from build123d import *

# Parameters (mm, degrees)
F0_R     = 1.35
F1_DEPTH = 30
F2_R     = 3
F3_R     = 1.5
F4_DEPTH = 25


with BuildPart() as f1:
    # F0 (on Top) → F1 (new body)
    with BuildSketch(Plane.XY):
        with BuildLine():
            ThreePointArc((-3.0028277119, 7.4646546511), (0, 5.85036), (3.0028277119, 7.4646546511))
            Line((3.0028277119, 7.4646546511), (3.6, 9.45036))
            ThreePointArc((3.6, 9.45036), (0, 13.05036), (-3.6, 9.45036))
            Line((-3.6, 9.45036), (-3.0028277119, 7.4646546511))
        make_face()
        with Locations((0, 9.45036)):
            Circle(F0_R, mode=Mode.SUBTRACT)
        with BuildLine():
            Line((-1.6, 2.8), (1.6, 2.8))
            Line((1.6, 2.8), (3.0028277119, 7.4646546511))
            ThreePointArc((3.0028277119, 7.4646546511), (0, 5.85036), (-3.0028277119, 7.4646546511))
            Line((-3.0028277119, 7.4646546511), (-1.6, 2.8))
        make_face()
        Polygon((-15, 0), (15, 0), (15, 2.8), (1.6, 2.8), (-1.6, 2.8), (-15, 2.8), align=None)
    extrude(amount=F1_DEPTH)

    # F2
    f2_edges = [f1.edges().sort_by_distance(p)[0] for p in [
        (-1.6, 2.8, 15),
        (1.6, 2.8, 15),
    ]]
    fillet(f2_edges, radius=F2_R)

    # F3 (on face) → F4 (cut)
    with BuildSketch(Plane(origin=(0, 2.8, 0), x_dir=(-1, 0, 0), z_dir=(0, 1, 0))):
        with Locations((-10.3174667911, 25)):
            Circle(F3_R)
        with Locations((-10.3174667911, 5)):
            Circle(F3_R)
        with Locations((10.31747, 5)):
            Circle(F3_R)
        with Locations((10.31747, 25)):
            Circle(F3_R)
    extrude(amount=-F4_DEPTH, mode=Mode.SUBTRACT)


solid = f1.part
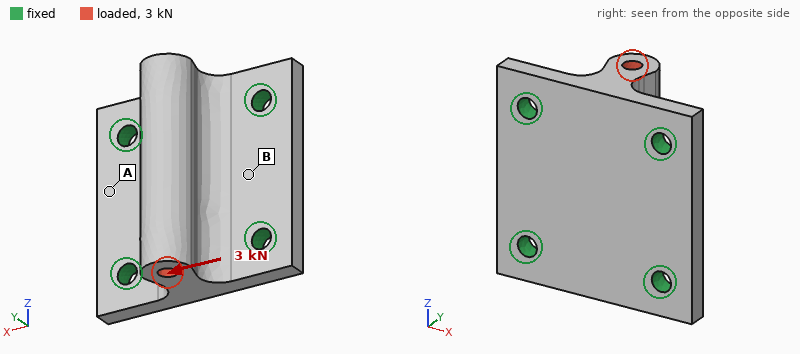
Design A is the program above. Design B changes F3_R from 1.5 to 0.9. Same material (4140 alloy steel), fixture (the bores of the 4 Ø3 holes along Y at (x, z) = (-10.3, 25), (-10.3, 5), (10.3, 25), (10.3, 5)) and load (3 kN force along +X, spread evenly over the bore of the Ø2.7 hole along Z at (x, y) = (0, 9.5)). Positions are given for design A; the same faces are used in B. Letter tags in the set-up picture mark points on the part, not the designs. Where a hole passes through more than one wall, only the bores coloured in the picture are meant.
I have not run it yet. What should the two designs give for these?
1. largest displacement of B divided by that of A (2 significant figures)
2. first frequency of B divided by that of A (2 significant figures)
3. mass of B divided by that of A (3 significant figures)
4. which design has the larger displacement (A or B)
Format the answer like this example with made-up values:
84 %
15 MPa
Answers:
1.1
0.88
1.01
B
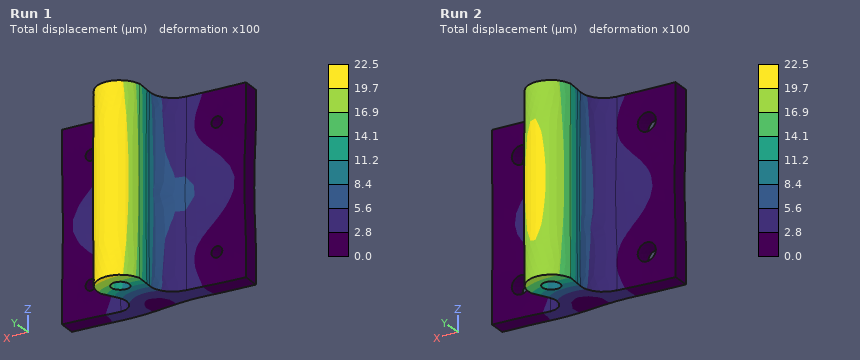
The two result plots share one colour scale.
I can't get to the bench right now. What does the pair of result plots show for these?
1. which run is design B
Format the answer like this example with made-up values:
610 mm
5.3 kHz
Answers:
Run 1
